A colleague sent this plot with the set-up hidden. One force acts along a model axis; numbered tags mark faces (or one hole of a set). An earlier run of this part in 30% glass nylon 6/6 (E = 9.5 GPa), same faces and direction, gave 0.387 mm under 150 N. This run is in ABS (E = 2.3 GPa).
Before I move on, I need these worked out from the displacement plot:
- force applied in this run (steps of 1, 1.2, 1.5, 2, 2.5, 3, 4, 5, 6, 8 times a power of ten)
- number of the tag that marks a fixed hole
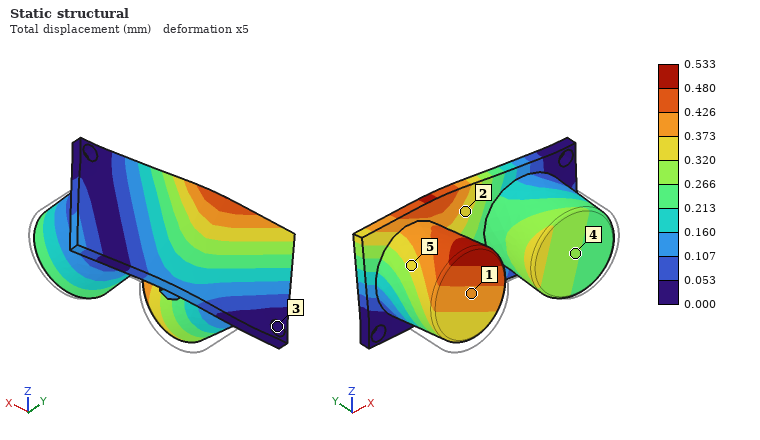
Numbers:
50 N
3
